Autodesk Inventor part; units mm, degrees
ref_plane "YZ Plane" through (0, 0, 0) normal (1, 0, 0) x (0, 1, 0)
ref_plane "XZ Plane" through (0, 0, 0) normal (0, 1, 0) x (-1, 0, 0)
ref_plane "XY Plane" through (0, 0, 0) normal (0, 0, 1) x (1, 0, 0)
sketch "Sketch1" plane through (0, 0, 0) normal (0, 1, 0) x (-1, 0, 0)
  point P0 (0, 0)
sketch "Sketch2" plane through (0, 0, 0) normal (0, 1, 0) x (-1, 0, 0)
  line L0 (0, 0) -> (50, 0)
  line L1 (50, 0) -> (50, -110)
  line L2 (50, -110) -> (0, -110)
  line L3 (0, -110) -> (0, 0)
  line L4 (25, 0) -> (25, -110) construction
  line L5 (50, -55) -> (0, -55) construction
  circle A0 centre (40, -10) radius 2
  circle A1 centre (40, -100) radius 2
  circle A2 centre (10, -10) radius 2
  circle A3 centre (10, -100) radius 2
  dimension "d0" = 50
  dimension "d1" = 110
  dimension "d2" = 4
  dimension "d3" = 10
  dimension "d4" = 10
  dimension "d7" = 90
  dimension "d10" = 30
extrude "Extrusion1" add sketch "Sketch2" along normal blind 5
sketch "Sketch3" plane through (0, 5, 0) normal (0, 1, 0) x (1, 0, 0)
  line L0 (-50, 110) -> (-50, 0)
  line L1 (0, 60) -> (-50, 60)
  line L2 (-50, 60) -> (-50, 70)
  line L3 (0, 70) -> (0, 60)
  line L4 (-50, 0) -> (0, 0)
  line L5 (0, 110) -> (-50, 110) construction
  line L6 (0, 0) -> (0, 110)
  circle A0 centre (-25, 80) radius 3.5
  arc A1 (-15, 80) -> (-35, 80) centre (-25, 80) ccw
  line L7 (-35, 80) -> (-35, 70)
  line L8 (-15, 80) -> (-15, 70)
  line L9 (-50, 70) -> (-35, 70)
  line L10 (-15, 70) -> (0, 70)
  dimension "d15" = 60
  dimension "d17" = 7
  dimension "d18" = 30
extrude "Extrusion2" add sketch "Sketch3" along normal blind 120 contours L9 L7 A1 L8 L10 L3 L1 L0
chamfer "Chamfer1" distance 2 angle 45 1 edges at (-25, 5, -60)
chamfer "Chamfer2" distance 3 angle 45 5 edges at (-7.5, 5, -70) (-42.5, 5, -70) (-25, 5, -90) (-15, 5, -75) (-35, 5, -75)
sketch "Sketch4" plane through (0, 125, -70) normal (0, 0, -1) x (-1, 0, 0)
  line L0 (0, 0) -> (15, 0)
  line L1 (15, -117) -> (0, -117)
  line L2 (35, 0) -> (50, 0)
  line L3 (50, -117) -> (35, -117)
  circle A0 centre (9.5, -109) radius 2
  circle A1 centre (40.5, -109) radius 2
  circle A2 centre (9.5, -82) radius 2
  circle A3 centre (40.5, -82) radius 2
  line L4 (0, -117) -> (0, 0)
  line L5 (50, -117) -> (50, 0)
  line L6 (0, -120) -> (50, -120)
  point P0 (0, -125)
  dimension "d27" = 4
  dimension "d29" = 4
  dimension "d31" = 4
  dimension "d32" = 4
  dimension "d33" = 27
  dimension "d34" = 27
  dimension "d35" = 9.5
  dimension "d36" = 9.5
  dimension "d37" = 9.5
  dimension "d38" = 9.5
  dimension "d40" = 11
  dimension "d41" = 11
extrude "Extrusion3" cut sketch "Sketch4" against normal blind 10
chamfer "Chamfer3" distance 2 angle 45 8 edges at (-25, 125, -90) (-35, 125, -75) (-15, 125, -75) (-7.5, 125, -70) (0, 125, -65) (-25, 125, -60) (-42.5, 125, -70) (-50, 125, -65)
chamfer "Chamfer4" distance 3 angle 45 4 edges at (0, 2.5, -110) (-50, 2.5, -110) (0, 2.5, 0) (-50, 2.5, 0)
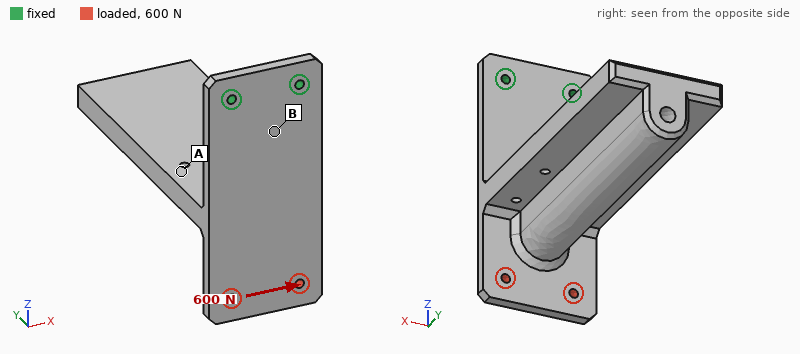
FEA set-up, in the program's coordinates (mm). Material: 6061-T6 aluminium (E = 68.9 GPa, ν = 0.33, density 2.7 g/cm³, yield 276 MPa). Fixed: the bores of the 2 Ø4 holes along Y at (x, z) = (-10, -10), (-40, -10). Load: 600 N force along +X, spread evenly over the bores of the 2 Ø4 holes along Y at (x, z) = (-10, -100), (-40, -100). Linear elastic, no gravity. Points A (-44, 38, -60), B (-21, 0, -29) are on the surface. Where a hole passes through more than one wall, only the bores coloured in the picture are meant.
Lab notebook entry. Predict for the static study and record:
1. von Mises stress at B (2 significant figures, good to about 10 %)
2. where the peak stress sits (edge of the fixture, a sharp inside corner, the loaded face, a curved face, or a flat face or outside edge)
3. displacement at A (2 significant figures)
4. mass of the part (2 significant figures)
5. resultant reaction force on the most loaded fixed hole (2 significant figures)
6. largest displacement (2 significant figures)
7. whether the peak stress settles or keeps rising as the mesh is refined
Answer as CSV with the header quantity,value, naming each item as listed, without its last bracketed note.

quantity,value
von Mises stress at B,8.6 MPa
where the peak stress sits,edge of the fixture
displacement at A,25 µm
mass of the part,340 g
resultant reaction force on the most loaded fixed hole,1.7 kN
largest displacement,69 µm
whether the peak stress settles or keeps rising as the mesh is refined,keeps rising
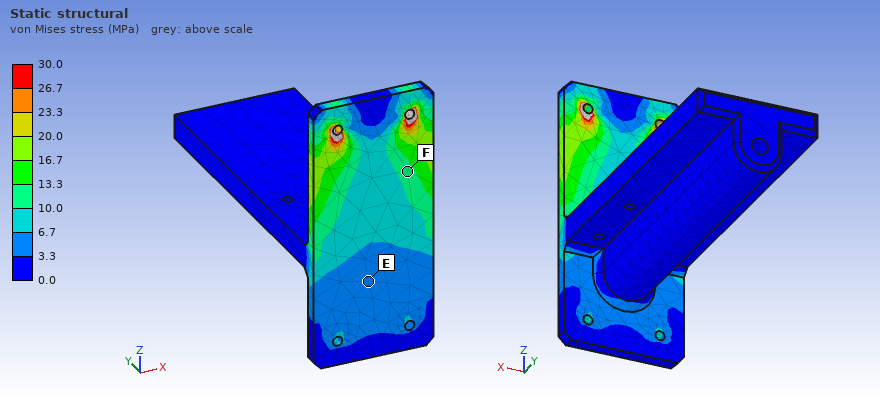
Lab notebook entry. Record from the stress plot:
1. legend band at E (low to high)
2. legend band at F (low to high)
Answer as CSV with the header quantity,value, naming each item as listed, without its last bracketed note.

quantity,value
legend band at E,3.3 to 6.7 MPa
legend band at F,10.0 to 13.3 MPa
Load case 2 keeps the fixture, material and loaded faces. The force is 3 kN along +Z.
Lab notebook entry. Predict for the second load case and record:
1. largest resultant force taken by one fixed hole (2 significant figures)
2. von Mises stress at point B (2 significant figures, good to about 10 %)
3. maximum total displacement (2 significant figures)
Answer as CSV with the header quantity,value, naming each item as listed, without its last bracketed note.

quantity,value
largest resultant force taken by one fixed hole,1.5 kN
von Mises stress at point B,11 MPa
maximum total displacement,26 µm
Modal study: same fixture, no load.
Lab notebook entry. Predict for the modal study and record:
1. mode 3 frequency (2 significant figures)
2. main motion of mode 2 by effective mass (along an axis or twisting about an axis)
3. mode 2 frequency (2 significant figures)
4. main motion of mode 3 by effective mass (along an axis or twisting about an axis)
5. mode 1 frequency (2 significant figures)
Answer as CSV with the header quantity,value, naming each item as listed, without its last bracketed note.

quantity,value
mode 3 frequency,560 Hz
main motion of mode 2 by effective mass,along X
mode 2 frequency,180 Hz
main motion of mode 3 by effective mass,along Y
mode 1 frequency,100 Hz
